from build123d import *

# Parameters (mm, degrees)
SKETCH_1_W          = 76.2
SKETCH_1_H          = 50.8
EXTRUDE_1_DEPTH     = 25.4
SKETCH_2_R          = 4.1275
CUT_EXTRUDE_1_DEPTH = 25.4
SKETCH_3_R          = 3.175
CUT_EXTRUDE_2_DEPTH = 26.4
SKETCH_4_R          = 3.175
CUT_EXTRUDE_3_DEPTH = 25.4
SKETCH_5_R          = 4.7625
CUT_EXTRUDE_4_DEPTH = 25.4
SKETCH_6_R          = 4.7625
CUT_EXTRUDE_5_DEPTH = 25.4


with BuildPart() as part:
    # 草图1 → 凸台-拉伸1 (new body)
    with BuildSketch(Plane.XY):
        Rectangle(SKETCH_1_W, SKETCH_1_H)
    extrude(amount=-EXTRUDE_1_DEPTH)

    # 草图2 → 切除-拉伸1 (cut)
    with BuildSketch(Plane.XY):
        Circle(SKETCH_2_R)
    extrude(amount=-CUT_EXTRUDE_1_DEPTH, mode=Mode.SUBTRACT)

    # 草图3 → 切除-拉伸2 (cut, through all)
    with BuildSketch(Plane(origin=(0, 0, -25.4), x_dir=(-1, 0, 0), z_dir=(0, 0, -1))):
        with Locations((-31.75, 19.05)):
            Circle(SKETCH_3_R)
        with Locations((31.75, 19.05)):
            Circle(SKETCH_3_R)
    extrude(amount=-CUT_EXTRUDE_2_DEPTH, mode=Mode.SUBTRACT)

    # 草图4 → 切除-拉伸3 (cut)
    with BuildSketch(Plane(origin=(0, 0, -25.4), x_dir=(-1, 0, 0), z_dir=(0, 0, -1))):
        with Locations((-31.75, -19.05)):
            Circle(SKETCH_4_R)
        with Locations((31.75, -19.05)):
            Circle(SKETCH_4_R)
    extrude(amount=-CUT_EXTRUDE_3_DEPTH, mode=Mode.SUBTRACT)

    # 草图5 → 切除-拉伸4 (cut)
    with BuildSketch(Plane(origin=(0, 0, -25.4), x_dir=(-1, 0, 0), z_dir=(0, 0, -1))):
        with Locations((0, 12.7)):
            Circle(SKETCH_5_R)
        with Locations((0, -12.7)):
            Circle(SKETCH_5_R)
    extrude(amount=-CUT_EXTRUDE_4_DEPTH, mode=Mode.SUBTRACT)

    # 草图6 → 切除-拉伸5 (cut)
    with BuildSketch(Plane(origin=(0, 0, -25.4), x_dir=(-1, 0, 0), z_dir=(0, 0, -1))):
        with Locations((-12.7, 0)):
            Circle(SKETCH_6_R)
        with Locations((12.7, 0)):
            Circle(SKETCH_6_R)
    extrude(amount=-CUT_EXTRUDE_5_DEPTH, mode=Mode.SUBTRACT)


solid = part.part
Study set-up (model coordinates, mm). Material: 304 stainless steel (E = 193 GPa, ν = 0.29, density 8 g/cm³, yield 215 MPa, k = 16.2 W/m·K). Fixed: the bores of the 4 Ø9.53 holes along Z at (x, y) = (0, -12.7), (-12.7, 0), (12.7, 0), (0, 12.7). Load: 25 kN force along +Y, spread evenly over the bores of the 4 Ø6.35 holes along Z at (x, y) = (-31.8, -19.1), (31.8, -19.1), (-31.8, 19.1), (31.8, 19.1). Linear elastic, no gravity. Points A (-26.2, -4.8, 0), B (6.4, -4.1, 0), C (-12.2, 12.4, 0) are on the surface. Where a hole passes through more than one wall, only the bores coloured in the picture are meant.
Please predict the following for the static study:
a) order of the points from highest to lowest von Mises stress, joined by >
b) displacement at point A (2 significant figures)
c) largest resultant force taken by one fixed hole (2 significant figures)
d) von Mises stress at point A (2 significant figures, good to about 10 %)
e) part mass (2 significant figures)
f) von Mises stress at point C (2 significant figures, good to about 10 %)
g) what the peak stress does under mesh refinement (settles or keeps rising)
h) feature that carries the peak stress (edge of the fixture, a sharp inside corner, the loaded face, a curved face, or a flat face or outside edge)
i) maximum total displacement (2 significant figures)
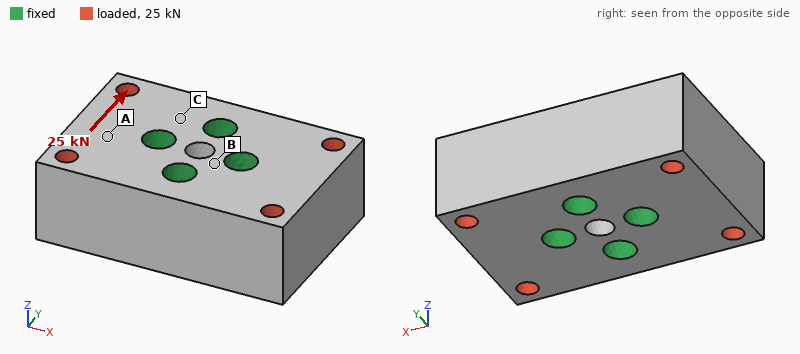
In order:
A > C > B
2.7 µm
12 kN
20 MPa
690 g
12 MPa
keeps rising
edge of the fixture
6.3 µm
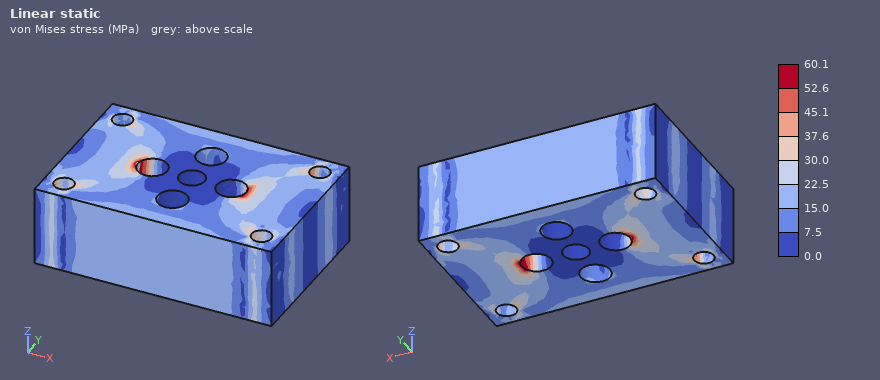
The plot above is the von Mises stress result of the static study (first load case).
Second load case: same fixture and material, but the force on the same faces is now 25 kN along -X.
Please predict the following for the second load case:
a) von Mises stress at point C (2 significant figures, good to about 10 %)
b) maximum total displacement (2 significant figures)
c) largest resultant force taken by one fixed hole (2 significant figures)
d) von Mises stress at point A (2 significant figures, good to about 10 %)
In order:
9.6 MPa
3.2 µm
7.7 kN
6.6 MPa
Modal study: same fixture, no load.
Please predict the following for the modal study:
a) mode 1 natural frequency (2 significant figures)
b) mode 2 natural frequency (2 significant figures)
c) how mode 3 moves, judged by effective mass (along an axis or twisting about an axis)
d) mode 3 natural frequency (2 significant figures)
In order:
19 kHz
19 kHz
twisting about Z
20 kHz
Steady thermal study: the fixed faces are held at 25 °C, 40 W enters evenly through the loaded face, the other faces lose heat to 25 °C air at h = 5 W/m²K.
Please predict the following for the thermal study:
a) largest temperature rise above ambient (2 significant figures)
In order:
30 K
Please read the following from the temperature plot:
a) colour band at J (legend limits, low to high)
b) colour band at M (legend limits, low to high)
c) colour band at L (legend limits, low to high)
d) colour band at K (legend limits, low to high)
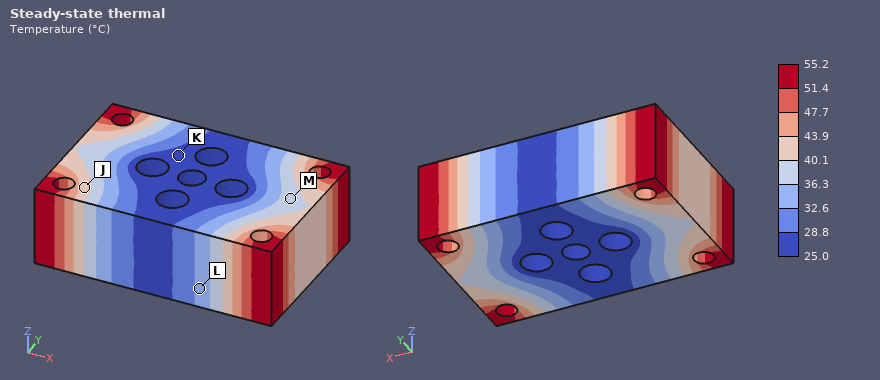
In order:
40.1 to 43.9 °C
36.3 to 40.1 °C
32.6 to 36.3 °C
25.0 to 28.8 °C
